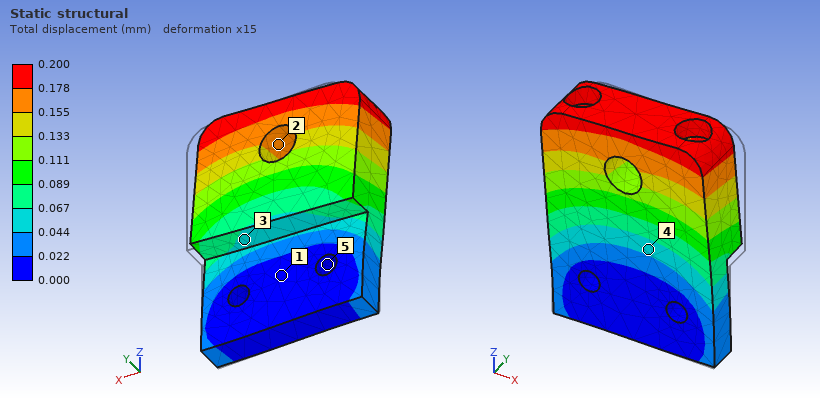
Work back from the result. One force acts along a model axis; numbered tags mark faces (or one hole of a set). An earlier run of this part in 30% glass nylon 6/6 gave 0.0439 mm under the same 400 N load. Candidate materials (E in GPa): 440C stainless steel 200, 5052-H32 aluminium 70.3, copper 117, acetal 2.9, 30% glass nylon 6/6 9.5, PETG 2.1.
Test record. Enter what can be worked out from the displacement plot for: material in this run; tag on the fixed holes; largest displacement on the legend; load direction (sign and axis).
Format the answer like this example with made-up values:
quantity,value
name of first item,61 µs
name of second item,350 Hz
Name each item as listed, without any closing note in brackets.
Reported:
quantity,value
material in this run,PETG
tag on the fixed holes,5
largest displacement on the legend,0.200 mm
load direction,-X
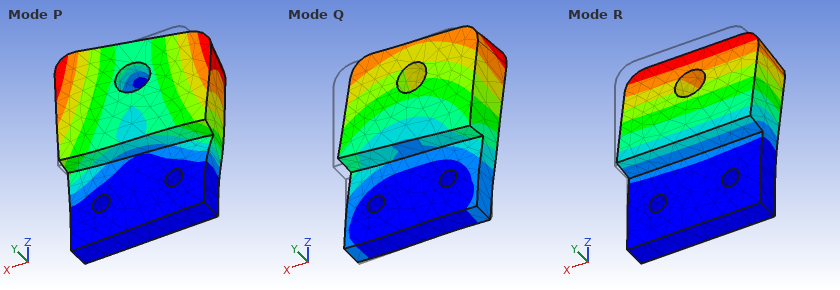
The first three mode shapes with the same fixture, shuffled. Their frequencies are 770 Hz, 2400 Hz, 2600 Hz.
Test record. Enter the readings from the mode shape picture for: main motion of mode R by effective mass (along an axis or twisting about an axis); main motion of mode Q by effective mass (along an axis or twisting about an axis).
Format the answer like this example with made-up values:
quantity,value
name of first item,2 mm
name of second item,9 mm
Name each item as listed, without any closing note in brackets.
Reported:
quantity,value
main motion of mode R by effective mass,along Y
main motion of mode Q by effective mass,along X
